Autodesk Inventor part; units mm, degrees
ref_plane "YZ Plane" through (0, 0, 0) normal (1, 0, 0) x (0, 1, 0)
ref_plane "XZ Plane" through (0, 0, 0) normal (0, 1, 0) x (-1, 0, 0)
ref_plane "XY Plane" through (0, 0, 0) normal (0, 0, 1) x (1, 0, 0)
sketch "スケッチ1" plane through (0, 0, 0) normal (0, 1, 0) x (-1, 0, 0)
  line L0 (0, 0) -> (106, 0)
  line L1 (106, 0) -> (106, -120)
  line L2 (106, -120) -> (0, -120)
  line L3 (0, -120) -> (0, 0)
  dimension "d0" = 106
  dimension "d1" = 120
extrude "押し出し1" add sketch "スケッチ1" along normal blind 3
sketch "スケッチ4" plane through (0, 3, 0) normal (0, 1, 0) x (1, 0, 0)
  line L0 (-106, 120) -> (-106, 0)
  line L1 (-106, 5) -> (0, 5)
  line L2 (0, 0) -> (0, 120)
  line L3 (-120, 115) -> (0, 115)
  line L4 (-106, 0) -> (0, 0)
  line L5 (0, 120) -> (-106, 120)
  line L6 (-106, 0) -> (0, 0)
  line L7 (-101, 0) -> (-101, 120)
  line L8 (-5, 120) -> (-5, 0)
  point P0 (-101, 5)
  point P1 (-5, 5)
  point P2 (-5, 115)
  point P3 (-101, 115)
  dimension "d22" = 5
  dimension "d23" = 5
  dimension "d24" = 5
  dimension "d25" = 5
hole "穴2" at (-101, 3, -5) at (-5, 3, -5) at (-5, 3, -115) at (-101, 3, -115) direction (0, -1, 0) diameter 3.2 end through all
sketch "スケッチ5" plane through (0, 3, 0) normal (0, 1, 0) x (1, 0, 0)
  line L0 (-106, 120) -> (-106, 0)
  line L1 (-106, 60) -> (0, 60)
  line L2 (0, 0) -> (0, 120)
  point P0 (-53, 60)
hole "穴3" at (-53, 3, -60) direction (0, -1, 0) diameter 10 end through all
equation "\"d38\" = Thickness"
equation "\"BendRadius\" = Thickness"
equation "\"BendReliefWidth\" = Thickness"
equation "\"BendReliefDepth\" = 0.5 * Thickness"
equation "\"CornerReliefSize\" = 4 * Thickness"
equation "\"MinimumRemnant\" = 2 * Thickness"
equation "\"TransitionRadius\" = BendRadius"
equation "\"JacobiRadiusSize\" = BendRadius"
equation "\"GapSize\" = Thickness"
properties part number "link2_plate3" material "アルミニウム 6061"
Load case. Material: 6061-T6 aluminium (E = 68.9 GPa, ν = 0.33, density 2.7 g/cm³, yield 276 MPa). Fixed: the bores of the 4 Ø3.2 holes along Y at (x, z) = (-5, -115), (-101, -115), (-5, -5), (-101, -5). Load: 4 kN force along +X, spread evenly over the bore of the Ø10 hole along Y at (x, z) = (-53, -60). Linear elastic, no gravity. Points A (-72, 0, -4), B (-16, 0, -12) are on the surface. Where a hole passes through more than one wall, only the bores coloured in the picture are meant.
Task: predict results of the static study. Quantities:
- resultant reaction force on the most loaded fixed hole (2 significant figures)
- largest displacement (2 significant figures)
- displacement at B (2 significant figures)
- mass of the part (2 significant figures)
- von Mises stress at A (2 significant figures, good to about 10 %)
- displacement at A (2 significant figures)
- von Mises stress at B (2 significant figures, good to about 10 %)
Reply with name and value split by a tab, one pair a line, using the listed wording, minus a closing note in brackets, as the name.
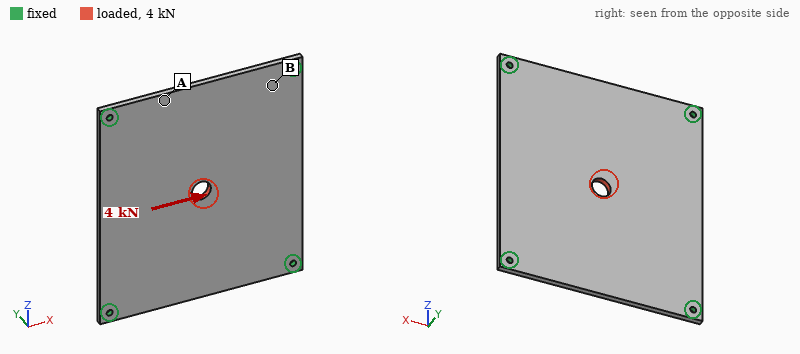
resultant reaction force on the most loaded fixed hole	1.2 kN
largest displacement	26 µm
displacement at B	5.8 µm
mass of the part	100 g
von Mises stress at A	7.6 MPa
displacement at A	6.8 µm
von Mises stress at B	19 MPa
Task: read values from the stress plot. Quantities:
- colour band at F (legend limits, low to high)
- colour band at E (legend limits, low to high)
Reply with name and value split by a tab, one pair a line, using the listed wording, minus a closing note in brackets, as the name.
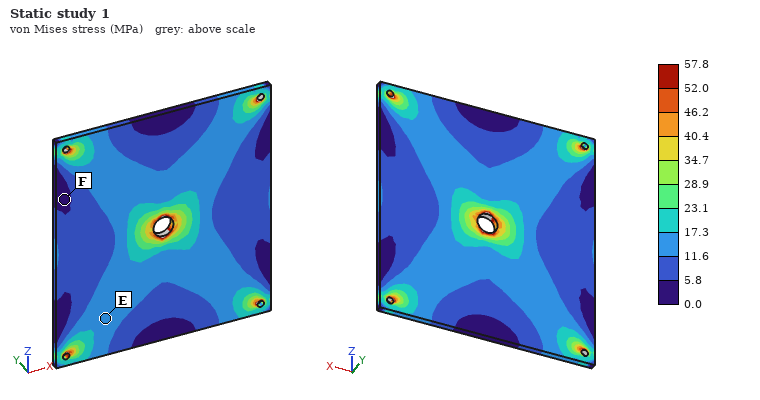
colour band at F	0.0 to 5.8 MPa
colour band at E	11.6 to 17.3 MPa
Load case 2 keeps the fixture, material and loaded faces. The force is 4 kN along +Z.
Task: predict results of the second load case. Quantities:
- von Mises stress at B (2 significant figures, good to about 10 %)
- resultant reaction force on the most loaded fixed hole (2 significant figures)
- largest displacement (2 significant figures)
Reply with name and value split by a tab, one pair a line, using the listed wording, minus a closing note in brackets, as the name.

von Mises stress at B	16 MPa
resultant reaction force on the most loaded fixed hole	1.1 kN
largest displacement	23 µm
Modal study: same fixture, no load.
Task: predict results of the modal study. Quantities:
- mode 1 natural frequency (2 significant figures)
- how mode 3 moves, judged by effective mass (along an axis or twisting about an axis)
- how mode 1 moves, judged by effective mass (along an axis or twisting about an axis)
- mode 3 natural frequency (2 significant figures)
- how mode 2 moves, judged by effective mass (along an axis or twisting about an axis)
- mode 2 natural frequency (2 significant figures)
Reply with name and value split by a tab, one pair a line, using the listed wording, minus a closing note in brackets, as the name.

mode 1 natural frequency	850 Hz
how mode 3 moves, judged by effective mass	twisting about X
how mode 1 moves, judged by effective mass	along Y
mode 3 natural frequency	1700 Hz
how mode 2 moves, judged by effective mass	twisting about Z
mode 2 natural frequency	1500 Hz
